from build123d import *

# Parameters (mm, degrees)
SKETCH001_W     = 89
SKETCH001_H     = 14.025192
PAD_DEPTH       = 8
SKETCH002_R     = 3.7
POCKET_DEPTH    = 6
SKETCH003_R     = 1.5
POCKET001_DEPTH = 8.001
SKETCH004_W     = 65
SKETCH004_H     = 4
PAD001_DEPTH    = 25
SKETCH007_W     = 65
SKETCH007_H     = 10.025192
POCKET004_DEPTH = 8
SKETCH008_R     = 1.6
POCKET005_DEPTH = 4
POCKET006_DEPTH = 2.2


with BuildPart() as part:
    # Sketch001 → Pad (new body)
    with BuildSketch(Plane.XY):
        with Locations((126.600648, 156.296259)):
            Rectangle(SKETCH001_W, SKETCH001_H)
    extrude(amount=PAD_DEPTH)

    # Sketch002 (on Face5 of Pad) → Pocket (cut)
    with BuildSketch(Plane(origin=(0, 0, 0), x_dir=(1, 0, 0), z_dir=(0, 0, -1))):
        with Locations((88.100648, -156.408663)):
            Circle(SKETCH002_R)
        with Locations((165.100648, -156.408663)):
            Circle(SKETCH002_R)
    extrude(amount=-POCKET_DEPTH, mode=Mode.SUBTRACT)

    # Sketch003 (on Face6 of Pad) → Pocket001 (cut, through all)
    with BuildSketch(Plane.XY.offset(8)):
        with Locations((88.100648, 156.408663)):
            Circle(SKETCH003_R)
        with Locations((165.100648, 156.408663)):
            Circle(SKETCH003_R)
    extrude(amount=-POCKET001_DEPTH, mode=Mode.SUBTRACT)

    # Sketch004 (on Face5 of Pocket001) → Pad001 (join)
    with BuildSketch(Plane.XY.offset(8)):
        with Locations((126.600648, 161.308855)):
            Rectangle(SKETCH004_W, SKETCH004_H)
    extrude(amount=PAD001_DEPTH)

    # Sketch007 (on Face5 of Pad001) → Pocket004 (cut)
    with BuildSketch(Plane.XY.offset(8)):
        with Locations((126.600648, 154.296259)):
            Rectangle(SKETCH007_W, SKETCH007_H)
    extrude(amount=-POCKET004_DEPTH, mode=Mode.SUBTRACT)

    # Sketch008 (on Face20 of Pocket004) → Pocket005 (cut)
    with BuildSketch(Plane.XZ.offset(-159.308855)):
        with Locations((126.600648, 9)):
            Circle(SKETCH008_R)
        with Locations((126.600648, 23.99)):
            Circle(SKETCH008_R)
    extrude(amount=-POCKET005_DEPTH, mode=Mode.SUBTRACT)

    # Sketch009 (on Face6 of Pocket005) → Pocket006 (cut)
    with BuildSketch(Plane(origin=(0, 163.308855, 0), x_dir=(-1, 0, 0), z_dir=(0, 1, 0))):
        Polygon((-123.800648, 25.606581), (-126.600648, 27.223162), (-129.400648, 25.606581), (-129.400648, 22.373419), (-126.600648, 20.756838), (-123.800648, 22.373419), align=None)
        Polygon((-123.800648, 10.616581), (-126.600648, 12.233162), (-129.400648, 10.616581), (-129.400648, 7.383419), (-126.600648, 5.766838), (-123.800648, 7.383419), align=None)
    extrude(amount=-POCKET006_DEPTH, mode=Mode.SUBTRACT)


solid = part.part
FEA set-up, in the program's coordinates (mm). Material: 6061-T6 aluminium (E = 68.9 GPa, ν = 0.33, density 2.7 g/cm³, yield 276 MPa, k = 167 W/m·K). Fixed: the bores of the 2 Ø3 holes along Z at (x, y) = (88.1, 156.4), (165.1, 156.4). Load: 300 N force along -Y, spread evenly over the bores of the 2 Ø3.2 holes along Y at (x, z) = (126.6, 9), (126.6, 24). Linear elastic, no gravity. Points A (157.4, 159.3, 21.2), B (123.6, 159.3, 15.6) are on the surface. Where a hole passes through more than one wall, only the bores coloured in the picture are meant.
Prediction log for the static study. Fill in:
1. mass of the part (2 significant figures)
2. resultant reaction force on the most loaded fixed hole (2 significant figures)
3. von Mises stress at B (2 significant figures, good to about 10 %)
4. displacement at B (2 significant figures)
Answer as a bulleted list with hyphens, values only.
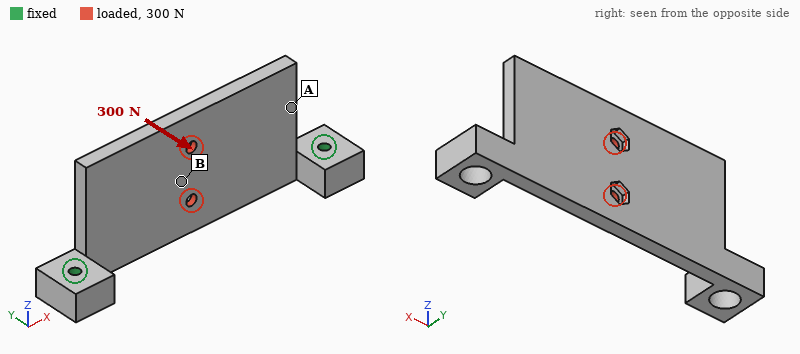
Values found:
- 29 g
- 290 N
- 38 MPa
- 0.15 mm
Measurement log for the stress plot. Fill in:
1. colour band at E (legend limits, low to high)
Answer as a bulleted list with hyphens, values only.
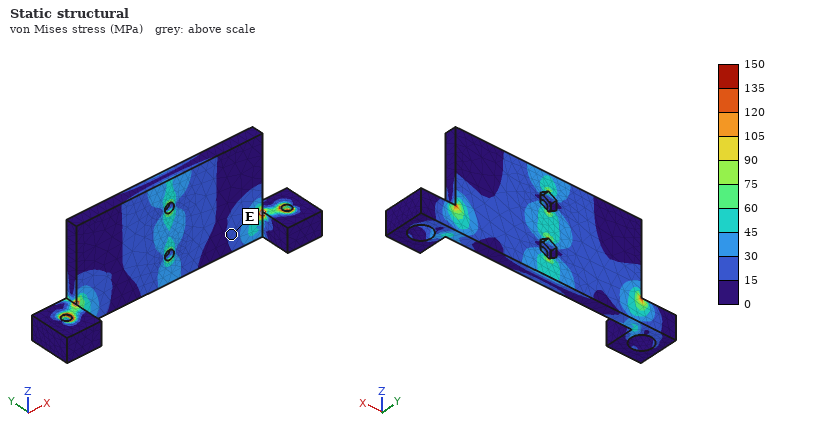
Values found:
- 15 to 30 MPa
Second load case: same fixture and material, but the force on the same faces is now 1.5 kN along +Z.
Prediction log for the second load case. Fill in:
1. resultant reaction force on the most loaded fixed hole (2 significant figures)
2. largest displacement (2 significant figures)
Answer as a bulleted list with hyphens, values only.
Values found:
- 750 N
- 82 µm
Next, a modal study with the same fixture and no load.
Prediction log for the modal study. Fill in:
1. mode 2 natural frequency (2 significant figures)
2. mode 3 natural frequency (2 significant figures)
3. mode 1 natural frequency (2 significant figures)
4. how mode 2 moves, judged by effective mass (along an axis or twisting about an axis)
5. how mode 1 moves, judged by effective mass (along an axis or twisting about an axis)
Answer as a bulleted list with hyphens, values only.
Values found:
- 3800 Hz
- 4100 Hz
- 1500 Hz
- along Y
- along Y
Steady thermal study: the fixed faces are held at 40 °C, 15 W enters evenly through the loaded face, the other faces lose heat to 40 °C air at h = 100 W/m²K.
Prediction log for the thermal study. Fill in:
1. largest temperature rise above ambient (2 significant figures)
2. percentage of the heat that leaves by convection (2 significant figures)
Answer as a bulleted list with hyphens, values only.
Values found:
- 21 K
- 47 %
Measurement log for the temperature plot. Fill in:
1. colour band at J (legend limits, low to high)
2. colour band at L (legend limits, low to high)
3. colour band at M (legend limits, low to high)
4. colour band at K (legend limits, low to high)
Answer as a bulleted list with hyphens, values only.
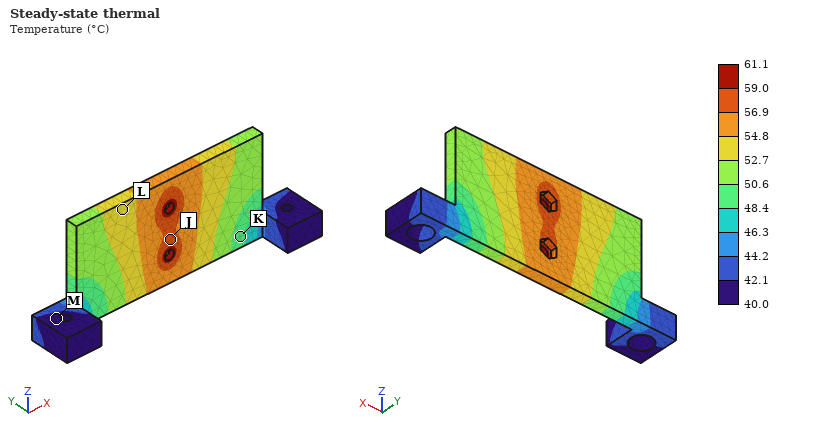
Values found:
- 56.9 to 59.0 °C
- 52.7 to 54.8 °C
- 40.0 to 42.1 °C
- 48.4 to 50.6 °C
